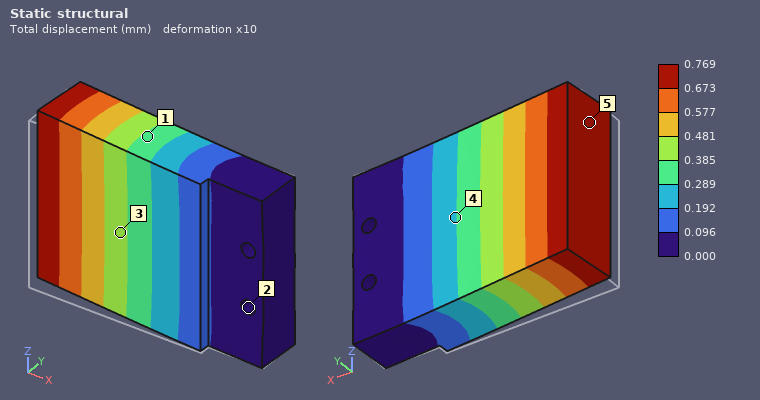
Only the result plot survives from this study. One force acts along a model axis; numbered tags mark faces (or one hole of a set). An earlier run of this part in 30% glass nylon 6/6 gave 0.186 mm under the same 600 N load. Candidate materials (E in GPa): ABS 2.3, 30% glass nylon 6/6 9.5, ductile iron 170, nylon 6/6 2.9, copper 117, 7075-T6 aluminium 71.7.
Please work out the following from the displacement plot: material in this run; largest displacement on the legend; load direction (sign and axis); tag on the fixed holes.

ABS
0.769 mm
+Y
2
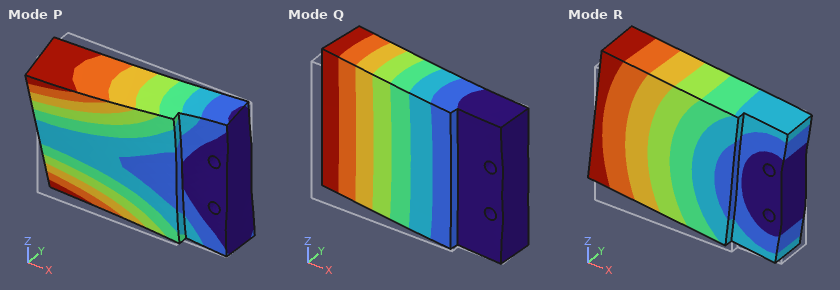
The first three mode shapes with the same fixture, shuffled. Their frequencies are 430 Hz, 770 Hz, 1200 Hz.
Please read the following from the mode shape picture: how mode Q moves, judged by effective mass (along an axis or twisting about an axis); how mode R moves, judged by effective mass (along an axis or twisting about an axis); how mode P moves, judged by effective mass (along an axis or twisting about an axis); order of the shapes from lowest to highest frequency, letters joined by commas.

along Y
along Z
twisting about X
Q, R, P
